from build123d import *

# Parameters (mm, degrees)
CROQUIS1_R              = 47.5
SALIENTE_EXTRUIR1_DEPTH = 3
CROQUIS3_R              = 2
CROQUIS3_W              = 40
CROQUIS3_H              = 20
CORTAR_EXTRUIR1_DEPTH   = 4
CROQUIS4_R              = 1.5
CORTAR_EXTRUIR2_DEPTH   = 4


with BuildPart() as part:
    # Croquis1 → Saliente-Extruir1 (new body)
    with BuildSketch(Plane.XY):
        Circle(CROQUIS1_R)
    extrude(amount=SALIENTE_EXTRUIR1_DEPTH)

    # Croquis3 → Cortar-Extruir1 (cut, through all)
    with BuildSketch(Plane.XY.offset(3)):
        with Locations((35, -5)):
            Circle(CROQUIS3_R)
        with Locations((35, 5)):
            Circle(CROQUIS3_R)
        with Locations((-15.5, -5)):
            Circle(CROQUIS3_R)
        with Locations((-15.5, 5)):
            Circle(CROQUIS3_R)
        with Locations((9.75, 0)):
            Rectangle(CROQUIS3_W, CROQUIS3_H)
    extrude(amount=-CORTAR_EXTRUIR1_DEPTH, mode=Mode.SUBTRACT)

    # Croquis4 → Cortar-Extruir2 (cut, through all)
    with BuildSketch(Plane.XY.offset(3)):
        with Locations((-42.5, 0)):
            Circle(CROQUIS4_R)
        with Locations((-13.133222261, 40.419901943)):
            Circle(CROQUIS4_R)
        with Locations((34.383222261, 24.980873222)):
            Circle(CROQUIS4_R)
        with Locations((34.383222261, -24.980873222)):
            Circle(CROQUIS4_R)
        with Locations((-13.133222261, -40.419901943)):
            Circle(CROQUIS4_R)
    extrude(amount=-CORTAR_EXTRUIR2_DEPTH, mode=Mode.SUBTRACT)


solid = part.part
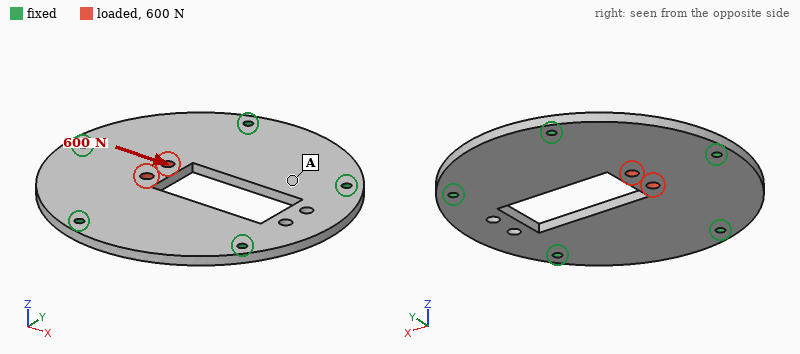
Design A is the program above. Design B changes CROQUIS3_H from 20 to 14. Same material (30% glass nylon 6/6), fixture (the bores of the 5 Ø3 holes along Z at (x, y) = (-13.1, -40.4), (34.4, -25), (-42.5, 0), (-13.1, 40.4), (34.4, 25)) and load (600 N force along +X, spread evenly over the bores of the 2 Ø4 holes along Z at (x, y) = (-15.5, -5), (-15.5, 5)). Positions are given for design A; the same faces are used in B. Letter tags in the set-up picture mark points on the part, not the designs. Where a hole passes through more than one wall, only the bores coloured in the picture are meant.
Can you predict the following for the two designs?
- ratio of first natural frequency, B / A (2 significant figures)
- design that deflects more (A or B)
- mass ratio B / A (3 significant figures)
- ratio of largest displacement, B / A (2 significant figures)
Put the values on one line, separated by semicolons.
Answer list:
0.94; A; 1.04; 0.89
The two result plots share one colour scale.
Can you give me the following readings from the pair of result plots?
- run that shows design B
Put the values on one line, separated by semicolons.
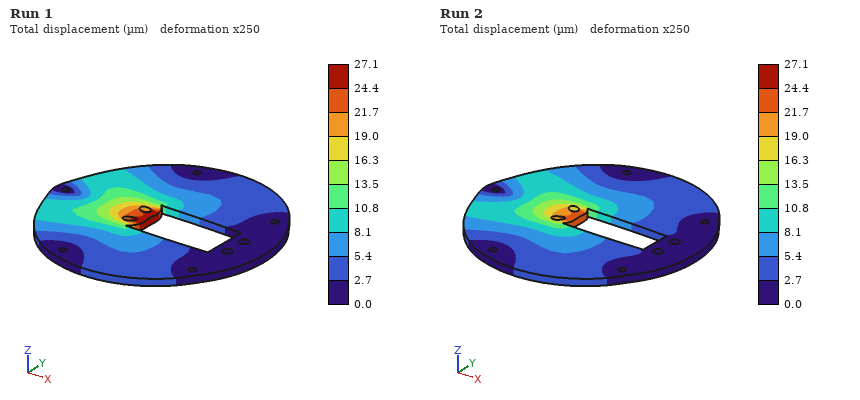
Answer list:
Run 2
